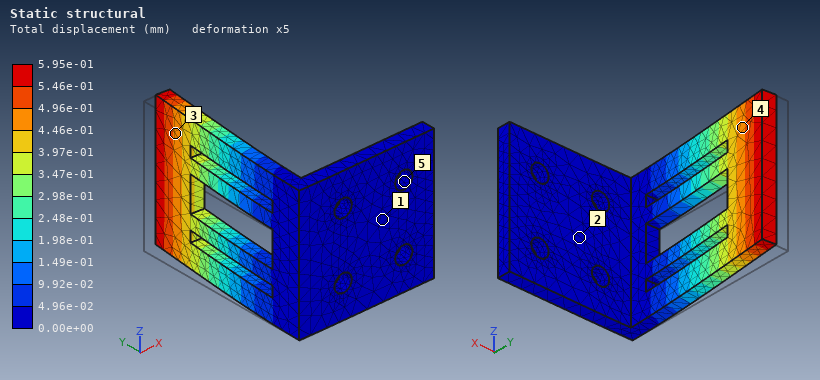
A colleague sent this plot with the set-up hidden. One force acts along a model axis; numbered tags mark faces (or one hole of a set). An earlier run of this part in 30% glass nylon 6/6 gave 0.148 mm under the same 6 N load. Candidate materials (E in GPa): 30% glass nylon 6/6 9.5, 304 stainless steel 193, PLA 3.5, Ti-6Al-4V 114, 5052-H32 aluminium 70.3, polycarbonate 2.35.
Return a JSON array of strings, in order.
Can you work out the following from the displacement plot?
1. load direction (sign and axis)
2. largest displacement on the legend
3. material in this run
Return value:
["+X", "5.95e-01 mm", "polycarbonate"]
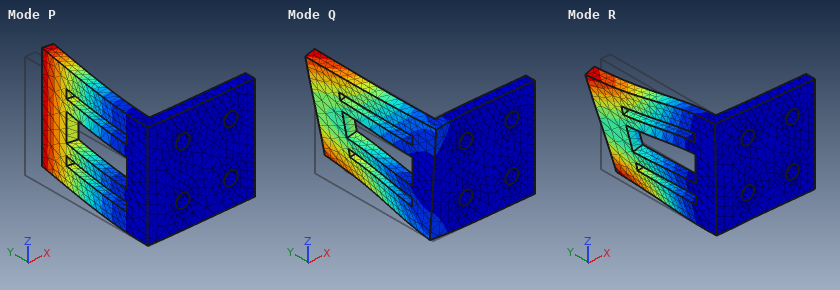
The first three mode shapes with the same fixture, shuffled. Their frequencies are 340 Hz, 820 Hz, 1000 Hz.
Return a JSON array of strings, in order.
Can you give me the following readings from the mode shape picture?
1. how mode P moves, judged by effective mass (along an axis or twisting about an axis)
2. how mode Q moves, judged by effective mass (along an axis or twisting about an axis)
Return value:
["along X", "along Z"]
